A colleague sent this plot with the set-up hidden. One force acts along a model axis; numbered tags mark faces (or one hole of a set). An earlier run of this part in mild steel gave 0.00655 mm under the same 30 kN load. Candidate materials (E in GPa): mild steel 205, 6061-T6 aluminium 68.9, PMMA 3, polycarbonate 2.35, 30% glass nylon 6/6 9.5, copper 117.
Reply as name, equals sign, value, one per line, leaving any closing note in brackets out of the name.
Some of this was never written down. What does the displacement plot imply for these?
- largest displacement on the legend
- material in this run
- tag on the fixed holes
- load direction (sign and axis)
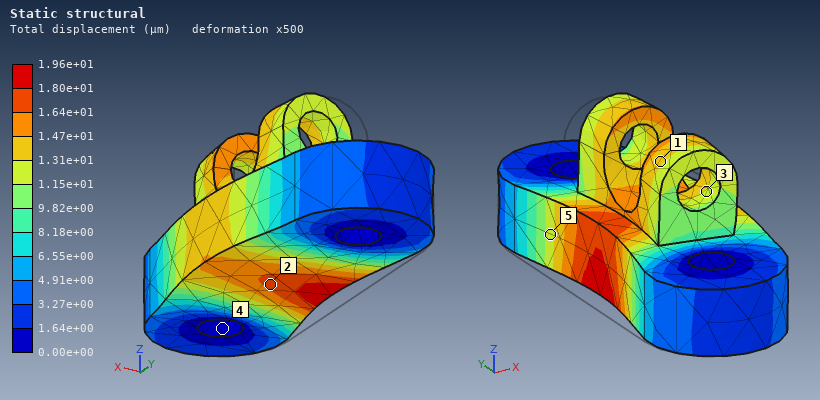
largest displacement on the legend = 1.96e+01 µm
material in this run = 6061-T6 aluminium
tag on the fixed holes = 4
load direction = +X
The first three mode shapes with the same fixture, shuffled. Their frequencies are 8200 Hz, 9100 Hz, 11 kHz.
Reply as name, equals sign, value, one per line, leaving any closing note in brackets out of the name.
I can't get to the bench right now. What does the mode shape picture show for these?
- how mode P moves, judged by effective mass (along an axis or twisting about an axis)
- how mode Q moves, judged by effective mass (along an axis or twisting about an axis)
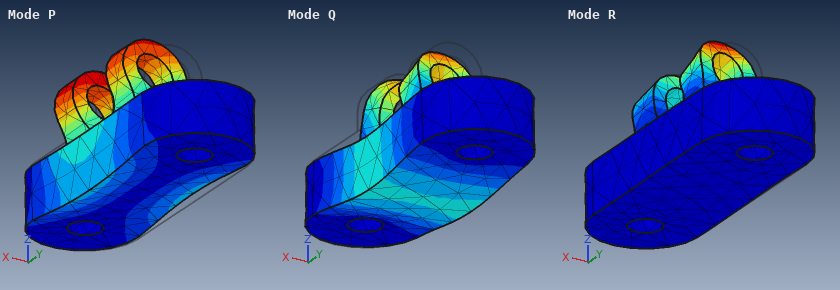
how mode P moves, judged by effective mass = along X
how mode Q moves, judged by effective mass = along Z
